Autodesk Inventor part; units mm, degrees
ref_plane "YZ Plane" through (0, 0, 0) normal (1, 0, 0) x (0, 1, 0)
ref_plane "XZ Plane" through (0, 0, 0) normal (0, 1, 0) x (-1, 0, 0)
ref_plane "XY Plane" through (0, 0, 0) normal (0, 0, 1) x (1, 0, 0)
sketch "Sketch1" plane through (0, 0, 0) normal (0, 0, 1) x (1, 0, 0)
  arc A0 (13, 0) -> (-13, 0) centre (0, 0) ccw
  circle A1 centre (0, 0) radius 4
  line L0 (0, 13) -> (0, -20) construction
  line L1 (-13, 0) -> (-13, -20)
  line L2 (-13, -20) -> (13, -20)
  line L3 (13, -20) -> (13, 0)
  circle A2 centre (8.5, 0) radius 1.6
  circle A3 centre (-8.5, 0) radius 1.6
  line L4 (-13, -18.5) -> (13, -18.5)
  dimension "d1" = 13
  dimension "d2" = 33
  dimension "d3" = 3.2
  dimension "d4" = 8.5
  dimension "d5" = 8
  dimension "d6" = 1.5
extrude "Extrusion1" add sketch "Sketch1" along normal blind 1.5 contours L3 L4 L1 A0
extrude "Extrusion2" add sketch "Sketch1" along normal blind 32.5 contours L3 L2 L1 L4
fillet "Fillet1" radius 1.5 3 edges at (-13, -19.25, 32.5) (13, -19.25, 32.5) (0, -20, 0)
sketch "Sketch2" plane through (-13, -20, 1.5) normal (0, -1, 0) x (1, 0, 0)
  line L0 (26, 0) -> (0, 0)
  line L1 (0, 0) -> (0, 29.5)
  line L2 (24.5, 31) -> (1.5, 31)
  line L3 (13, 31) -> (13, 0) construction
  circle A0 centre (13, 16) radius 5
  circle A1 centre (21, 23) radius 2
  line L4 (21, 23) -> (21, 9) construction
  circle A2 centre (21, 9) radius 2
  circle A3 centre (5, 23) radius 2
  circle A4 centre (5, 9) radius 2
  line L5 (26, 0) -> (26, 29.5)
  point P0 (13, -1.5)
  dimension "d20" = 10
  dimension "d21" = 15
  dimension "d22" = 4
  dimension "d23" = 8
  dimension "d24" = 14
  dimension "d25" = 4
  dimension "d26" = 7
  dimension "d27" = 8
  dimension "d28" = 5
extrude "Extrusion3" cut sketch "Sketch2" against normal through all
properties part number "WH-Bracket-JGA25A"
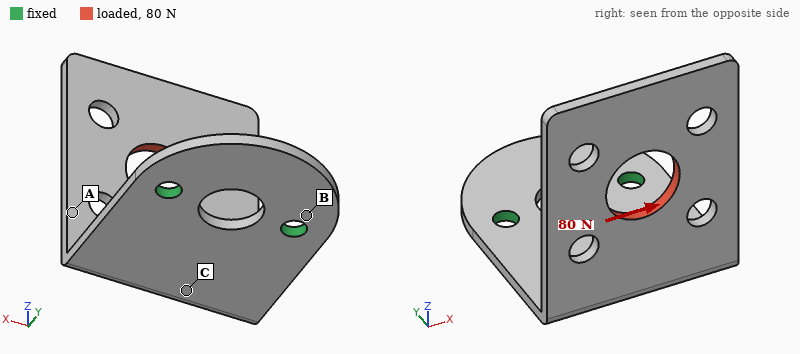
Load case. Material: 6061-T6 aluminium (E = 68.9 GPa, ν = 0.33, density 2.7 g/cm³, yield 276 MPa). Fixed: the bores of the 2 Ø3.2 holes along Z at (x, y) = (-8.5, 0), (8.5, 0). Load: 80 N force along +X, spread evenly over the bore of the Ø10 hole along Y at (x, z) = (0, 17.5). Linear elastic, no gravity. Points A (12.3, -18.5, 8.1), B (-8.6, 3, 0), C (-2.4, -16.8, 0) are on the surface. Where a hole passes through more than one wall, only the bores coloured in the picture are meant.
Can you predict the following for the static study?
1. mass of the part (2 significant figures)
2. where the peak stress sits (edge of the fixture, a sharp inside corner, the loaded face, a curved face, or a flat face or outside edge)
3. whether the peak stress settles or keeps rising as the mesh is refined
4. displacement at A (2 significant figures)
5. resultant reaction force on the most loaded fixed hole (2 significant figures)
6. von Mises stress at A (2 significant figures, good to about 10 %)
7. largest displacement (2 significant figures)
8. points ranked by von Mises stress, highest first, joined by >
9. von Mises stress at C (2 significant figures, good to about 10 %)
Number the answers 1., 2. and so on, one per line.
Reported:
1. 5.6 g
2. edge of the fixture
3. keeps rising
4. 0.26 mm
5. 110 N
6. 36 MPa
7. 0.62 mm
8. C > A > B
9. 68 MPa
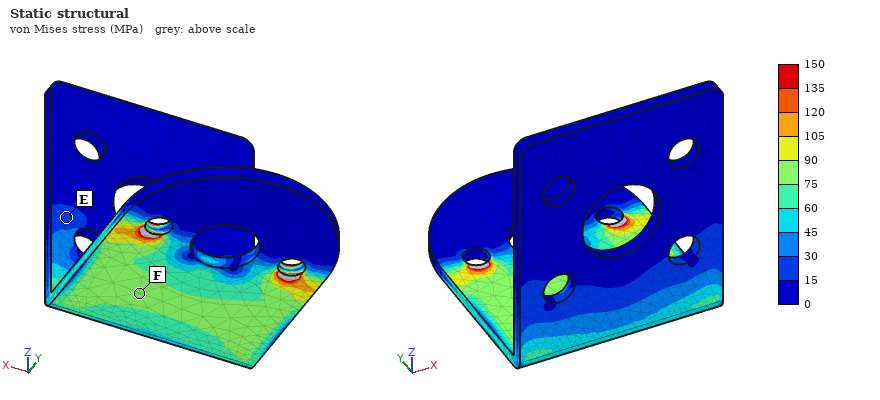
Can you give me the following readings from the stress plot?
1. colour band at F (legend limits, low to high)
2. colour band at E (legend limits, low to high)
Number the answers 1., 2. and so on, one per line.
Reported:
1. 75 to 90 MPa
2. 15 to 30 MPa
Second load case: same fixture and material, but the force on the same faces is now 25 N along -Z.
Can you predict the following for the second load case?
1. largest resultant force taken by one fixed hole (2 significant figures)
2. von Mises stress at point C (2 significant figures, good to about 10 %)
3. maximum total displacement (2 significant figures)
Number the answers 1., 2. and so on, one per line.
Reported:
1. 13 N
2. 6.9 MPa
3. 0.31 mm
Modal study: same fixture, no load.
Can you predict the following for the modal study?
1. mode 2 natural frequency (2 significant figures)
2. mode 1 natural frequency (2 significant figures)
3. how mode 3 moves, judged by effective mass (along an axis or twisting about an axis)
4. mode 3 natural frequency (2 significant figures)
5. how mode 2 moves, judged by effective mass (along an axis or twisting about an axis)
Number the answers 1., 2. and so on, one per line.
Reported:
1. 1300 Hz
2. 640 Hz
3. along Z
4. 1900 Hz
5. along X
